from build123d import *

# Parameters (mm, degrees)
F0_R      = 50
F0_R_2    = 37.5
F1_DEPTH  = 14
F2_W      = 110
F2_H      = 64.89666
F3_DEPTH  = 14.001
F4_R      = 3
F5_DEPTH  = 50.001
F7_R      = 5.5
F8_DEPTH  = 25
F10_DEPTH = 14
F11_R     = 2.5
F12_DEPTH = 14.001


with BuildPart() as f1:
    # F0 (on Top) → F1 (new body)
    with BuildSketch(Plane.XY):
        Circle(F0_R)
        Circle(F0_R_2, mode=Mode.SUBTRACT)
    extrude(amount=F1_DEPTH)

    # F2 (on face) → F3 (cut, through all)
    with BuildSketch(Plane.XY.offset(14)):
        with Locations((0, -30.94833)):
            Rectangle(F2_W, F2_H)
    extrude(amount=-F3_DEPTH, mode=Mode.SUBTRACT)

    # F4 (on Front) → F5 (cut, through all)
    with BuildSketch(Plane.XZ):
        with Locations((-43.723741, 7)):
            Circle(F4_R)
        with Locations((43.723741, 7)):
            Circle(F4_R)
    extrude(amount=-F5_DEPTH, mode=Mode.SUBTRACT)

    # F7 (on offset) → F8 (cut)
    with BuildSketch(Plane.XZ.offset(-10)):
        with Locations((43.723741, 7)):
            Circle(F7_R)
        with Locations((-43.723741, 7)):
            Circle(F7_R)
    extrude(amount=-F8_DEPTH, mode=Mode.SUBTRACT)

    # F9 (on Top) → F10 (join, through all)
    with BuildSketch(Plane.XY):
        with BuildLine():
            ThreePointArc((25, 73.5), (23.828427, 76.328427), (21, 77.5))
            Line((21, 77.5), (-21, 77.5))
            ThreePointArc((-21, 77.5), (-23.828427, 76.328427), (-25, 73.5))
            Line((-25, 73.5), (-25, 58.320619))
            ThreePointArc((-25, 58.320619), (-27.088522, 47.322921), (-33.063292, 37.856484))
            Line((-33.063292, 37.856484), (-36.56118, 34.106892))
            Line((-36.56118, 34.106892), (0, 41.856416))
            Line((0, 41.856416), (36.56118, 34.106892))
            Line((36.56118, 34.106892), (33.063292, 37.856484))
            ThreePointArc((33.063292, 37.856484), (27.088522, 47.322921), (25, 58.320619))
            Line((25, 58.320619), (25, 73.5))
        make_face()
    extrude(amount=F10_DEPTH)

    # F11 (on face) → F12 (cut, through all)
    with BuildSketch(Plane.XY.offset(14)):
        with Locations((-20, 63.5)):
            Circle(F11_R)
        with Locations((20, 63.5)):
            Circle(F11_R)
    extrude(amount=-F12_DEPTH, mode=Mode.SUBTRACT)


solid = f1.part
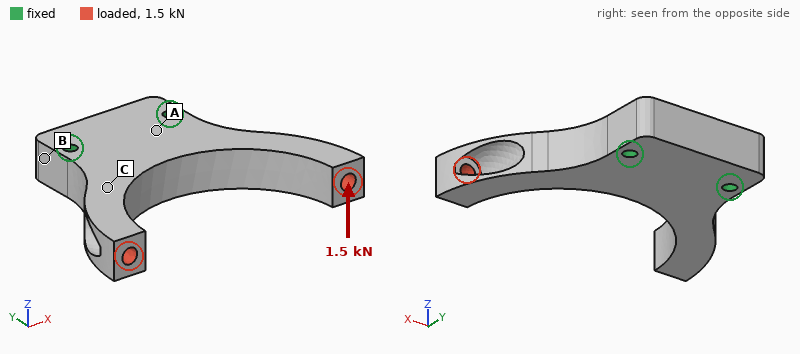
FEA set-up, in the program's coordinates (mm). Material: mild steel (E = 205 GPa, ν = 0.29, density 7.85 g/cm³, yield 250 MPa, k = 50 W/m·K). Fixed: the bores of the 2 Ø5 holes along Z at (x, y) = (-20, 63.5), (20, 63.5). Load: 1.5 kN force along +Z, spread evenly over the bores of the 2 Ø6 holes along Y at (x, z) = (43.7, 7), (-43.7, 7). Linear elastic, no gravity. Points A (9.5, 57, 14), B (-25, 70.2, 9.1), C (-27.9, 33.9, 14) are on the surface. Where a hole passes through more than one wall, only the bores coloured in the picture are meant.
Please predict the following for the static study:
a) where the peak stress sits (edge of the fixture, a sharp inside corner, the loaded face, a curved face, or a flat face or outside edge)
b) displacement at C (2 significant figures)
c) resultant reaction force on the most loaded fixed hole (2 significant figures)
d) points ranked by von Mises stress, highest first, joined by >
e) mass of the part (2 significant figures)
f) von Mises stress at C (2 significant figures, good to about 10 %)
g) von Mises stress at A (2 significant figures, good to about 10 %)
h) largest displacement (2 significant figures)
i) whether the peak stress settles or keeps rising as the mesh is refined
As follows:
edge of the fixture
0.024 mm
750 N
C > A > B
330 g
58 MPa
27 MPa
0.10 mm
keeps rising
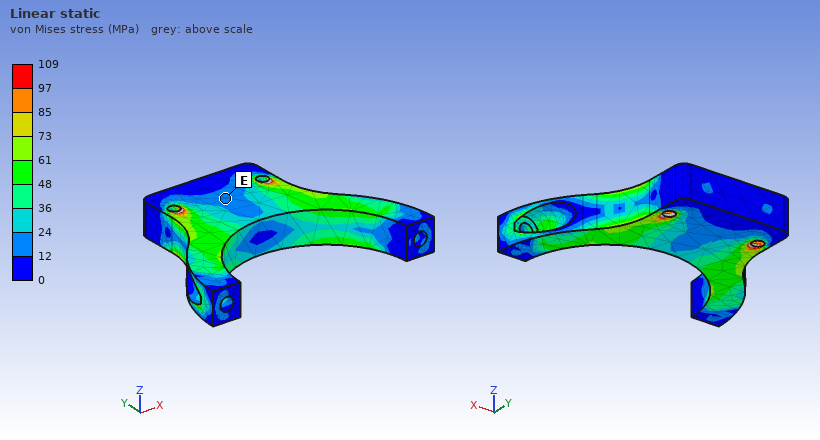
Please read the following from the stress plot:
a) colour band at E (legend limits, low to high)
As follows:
12 to 24 MPa
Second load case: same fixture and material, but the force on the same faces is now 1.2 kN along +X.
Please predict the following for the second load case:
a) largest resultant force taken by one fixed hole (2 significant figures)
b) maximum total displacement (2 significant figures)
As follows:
1.8 kN
47 µm
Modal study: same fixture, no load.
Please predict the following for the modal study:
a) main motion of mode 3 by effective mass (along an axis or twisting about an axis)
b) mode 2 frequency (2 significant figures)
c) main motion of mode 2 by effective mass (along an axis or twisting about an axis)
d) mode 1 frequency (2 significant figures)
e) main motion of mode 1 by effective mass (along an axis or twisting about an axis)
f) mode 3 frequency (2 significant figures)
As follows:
along X
3600 Hz
twisting about Y
3400 Hz
along Z
4800 Hz
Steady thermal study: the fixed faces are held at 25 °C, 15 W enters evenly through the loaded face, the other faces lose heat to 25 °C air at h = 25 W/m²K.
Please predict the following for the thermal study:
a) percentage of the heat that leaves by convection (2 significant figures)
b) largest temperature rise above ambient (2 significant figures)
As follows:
31 %
51 K
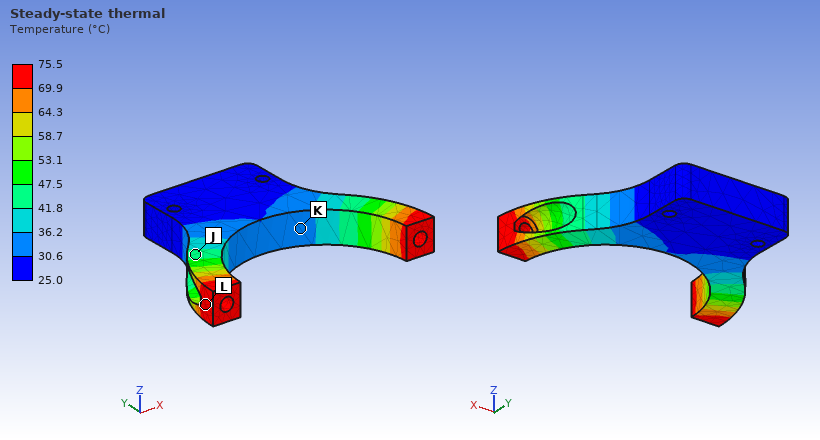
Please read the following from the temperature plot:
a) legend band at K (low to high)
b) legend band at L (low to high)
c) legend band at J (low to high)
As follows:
30.6 to 36.2 °C
69.9 to 75.5 °C
41.8 to 47.5 °C
